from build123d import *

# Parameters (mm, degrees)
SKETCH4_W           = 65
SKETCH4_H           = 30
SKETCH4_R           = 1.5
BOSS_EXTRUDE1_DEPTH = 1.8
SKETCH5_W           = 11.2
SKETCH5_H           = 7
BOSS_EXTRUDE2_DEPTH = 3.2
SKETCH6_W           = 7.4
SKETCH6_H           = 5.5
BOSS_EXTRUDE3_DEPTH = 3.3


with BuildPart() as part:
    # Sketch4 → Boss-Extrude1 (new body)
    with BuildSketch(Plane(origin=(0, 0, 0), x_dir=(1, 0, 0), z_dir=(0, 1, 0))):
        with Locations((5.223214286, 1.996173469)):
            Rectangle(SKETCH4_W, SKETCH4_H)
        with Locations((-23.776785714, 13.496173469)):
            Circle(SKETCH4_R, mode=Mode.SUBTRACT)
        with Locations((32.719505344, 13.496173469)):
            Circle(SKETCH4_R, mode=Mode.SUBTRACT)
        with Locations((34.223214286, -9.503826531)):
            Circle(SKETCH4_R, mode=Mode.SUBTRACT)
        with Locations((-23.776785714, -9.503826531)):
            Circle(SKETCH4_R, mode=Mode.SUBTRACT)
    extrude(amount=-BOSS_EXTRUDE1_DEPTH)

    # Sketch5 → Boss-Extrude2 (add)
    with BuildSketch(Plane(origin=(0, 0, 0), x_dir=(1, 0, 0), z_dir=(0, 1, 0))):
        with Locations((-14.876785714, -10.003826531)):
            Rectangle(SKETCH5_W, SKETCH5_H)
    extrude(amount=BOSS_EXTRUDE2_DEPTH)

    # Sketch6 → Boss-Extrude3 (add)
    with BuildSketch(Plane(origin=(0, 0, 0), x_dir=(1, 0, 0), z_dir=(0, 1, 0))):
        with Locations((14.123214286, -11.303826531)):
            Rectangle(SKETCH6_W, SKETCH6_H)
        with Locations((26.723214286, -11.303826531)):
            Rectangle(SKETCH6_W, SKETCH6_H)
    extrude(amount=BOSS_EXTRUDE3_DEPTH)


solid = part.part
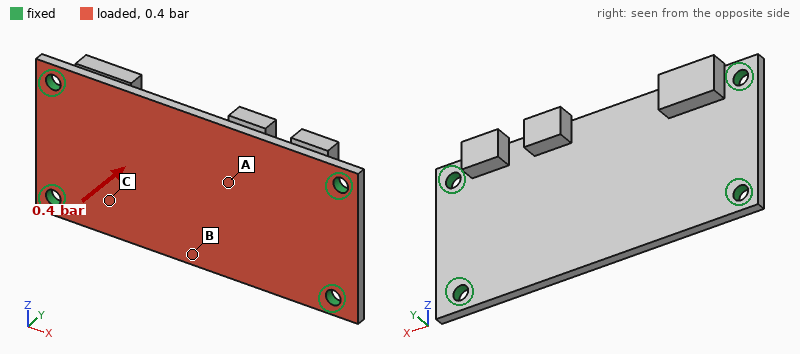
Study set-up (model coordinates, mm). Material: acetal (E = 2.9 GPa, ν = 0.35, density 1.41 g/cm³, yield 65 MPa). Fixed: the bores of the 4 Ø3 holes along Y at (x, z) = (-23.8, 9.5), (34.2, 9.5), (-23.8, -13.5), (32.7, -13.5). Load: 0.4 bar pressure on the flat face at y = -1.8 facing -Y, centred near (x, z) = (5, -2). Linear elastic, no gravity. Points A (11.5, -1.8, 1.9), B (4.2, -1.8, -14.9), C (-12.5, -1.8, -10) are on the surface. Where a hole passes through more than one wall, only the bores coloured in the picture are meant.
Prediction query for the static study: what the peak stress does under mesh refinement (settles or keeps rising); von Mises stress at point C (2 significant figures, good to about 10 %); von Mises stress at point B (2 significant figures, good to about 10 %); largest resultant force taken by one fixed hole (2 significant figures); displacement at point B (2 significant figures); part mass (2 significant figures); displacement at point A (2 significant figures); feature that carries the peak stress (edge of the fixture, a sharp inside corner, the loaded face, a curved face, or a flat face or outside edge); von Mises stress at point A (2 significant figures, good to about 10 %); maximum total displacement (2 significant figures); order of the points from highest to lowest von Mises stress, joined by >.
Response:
keeps rising
2.5 MPa
10 MPa
21 N
0.78 mm
5.6 g
0.65 mm
edge of the fixture
6.6 MPa
0.80 mm
B > A > C
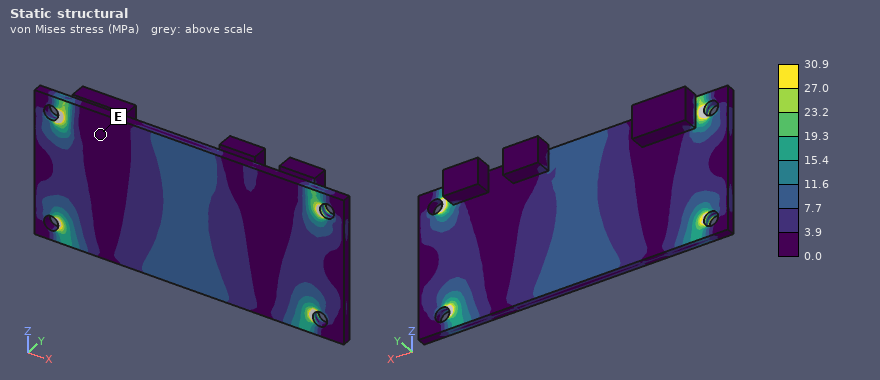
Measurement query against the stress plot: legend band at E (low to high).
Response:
0.0 to 3.9 MPa
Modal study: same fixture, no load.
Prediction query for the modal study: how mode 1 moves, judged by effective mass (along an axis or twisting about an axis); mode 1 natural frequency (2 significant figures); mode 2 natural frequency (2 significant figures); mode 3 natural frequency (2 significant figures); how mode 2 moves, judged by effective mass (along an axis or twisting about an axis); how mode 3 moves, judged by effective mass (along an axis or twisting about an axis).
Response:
along Y
800 Hz
1300 Hz
2100 Hz
twisting about X
twisting about Z
